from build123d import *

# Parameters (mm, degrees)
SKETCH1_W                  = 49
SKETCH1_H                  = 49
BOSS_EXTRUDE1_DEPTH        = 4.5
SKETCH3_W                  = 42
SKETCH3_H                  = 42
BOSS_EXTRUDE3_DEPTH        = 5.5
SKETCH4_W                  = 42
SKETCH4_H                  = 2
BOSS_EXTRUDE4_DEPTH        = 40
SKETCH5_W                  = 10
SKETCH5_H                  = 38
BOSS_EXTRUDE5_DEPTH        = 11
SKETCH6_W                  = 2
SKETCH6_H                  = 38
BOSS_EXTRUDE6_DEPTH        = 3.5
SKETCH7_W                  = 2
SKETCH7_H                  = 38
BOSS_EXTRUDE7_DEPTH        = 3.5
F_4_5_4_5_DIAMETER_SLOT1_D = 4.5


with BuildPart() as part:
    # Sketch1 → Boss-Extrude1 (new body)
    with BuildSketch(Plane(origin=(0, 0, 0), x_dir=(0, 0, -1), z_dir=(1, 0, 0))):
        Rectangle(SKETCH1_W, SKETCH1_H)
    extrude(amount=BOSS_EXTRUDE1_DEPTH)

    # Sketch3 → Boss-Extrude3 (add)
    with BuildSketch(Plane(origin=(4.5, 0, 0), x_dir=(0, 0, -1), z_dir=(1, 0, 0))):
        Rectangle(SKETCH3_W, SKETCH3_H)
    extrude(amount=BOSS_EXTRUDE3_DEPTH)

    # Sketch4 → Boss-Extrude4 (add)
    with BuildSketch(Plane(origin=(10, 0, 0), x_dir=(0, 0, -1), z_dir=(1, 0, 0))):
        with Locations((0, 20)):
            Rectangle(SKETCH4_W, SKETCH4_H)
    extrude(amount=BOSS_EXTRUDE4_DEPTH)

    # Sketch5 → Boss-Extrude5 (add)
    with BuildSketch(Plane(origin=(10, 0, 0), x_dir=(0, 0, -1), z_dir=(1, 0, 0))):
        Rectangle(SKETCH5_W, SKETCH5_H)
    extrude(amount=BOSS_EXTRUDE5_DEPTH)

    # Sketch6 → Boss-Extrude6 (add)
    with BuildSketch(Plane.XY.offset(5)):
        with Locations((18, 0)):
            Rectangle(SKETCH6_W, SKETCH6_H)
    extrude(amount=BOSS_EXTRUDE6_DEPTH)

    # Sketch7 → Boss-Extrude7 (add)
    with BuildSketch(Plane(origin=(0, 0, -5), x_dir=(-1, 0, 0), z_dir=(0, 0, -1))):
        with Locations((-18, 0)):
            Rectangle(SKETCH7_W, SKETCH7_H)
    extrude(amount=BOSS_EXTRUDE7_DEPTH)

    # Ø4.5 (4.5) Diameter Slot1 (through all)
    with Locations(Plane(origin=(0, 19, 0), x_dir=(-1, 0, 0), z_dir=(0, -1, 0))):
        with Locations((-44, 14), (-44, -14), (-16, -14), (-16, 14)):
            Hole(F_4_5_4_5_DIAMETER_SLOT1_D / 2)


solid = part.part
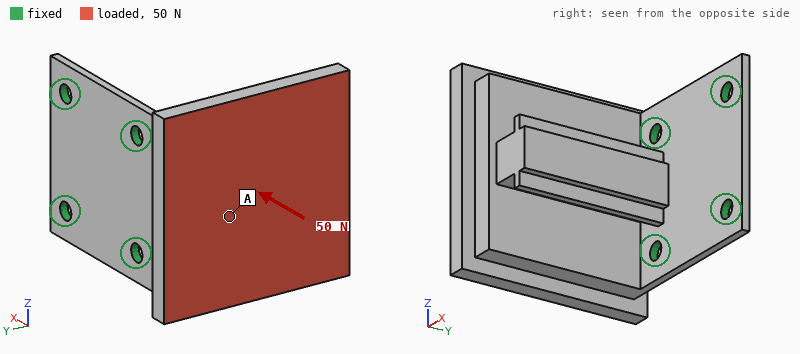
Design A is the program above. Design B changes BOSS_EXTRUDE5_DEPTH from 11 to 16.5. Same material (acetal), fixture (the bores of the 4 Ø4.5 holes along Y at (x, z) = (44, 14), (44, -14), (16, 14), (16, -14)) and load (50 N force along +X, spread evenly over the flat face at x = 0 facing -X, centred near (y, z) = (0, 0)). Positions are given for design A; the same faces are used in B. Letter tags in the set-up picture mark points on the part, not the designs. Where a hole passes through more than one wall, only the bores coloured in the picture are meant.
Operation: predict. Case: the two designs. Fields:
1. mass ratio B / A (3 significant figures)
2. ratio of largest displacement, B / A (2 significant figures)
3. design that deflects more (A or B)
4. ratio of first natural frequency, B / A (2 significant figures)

1.07
0.66
A
1.2
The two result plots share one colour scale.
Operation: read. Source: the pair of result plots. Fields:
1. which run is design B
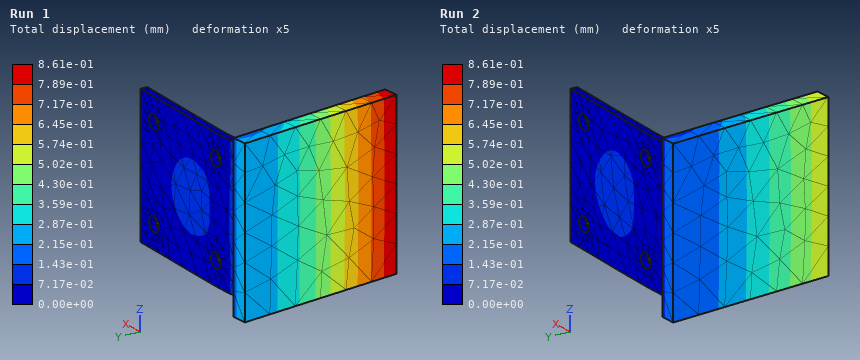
Run 2
